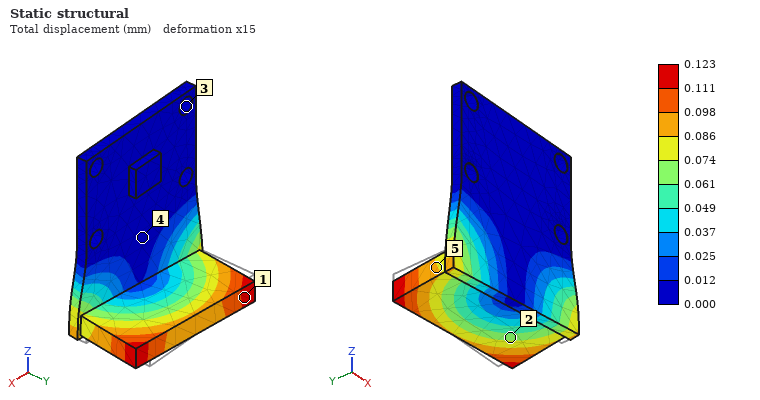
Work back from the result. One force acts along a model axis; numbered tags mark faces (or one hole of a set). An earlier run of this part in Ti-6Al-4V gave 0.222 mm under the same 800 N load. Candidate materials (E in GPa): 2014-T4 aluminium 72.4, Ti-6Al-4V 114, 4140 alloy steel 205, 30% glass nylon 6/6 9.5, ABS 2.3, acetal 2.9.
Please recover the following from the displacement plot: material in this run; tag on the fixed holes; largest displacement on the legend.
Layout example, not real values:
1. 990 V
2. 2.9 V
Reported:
1. 4140 alloy steel
2. 3
3. 0.123 mm
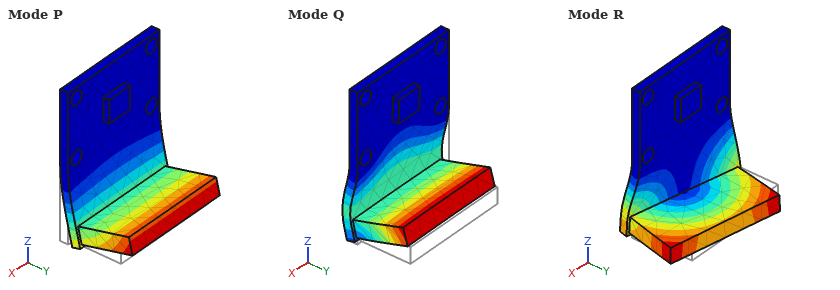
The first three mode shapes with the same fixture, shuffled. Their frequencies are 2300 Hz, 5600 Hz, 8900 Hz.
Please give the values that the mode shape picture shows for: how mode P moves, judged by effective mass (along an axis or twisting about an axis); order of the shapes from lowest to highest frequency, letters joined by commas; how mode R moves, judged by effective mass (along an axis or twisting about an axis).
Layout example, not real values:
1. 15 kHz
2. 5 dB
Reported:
1. along Y
2. P, R, Q
3. along X
